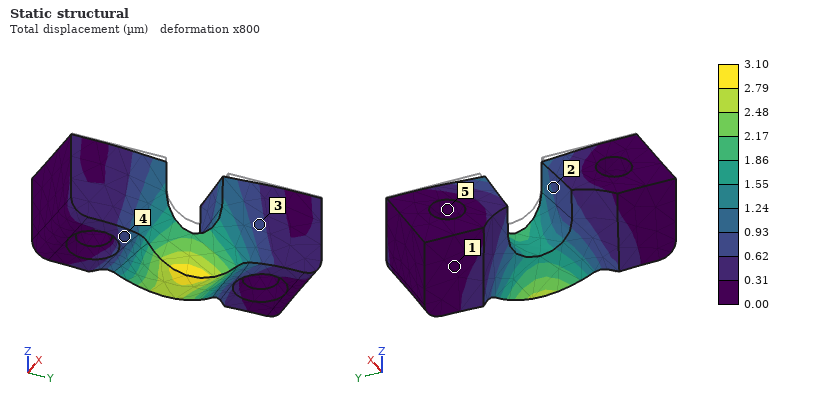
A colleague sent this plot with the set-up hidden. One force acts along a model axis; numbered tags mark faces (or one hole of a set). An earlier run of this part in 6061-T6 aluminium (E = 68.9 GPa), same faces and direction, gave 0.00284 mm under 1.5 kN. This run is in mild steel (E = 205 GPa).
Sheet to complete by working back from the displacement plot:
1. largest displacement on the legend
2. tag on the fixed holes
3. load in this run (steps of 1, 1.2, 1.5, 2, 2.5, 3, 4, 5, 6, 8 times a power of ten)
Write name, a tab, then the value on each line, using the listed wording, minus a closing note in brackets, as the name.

largest displacement on the legend	3.10 µm
tag on the fixed holes	5
load in this run	5 kN
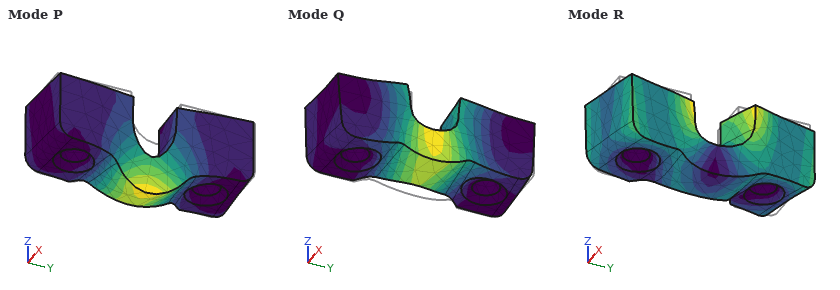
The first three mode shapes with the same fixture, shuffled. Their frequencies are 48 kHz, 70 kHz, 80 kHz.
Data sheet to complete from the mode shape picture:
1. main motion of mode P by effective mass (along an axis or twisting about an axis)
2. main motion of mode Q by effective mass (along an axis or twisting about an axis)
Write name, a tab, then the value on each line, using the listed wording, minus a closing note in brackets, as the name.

main motion of mode P by effective mass	along X
main motion of mode Q by effective mass	along Z
